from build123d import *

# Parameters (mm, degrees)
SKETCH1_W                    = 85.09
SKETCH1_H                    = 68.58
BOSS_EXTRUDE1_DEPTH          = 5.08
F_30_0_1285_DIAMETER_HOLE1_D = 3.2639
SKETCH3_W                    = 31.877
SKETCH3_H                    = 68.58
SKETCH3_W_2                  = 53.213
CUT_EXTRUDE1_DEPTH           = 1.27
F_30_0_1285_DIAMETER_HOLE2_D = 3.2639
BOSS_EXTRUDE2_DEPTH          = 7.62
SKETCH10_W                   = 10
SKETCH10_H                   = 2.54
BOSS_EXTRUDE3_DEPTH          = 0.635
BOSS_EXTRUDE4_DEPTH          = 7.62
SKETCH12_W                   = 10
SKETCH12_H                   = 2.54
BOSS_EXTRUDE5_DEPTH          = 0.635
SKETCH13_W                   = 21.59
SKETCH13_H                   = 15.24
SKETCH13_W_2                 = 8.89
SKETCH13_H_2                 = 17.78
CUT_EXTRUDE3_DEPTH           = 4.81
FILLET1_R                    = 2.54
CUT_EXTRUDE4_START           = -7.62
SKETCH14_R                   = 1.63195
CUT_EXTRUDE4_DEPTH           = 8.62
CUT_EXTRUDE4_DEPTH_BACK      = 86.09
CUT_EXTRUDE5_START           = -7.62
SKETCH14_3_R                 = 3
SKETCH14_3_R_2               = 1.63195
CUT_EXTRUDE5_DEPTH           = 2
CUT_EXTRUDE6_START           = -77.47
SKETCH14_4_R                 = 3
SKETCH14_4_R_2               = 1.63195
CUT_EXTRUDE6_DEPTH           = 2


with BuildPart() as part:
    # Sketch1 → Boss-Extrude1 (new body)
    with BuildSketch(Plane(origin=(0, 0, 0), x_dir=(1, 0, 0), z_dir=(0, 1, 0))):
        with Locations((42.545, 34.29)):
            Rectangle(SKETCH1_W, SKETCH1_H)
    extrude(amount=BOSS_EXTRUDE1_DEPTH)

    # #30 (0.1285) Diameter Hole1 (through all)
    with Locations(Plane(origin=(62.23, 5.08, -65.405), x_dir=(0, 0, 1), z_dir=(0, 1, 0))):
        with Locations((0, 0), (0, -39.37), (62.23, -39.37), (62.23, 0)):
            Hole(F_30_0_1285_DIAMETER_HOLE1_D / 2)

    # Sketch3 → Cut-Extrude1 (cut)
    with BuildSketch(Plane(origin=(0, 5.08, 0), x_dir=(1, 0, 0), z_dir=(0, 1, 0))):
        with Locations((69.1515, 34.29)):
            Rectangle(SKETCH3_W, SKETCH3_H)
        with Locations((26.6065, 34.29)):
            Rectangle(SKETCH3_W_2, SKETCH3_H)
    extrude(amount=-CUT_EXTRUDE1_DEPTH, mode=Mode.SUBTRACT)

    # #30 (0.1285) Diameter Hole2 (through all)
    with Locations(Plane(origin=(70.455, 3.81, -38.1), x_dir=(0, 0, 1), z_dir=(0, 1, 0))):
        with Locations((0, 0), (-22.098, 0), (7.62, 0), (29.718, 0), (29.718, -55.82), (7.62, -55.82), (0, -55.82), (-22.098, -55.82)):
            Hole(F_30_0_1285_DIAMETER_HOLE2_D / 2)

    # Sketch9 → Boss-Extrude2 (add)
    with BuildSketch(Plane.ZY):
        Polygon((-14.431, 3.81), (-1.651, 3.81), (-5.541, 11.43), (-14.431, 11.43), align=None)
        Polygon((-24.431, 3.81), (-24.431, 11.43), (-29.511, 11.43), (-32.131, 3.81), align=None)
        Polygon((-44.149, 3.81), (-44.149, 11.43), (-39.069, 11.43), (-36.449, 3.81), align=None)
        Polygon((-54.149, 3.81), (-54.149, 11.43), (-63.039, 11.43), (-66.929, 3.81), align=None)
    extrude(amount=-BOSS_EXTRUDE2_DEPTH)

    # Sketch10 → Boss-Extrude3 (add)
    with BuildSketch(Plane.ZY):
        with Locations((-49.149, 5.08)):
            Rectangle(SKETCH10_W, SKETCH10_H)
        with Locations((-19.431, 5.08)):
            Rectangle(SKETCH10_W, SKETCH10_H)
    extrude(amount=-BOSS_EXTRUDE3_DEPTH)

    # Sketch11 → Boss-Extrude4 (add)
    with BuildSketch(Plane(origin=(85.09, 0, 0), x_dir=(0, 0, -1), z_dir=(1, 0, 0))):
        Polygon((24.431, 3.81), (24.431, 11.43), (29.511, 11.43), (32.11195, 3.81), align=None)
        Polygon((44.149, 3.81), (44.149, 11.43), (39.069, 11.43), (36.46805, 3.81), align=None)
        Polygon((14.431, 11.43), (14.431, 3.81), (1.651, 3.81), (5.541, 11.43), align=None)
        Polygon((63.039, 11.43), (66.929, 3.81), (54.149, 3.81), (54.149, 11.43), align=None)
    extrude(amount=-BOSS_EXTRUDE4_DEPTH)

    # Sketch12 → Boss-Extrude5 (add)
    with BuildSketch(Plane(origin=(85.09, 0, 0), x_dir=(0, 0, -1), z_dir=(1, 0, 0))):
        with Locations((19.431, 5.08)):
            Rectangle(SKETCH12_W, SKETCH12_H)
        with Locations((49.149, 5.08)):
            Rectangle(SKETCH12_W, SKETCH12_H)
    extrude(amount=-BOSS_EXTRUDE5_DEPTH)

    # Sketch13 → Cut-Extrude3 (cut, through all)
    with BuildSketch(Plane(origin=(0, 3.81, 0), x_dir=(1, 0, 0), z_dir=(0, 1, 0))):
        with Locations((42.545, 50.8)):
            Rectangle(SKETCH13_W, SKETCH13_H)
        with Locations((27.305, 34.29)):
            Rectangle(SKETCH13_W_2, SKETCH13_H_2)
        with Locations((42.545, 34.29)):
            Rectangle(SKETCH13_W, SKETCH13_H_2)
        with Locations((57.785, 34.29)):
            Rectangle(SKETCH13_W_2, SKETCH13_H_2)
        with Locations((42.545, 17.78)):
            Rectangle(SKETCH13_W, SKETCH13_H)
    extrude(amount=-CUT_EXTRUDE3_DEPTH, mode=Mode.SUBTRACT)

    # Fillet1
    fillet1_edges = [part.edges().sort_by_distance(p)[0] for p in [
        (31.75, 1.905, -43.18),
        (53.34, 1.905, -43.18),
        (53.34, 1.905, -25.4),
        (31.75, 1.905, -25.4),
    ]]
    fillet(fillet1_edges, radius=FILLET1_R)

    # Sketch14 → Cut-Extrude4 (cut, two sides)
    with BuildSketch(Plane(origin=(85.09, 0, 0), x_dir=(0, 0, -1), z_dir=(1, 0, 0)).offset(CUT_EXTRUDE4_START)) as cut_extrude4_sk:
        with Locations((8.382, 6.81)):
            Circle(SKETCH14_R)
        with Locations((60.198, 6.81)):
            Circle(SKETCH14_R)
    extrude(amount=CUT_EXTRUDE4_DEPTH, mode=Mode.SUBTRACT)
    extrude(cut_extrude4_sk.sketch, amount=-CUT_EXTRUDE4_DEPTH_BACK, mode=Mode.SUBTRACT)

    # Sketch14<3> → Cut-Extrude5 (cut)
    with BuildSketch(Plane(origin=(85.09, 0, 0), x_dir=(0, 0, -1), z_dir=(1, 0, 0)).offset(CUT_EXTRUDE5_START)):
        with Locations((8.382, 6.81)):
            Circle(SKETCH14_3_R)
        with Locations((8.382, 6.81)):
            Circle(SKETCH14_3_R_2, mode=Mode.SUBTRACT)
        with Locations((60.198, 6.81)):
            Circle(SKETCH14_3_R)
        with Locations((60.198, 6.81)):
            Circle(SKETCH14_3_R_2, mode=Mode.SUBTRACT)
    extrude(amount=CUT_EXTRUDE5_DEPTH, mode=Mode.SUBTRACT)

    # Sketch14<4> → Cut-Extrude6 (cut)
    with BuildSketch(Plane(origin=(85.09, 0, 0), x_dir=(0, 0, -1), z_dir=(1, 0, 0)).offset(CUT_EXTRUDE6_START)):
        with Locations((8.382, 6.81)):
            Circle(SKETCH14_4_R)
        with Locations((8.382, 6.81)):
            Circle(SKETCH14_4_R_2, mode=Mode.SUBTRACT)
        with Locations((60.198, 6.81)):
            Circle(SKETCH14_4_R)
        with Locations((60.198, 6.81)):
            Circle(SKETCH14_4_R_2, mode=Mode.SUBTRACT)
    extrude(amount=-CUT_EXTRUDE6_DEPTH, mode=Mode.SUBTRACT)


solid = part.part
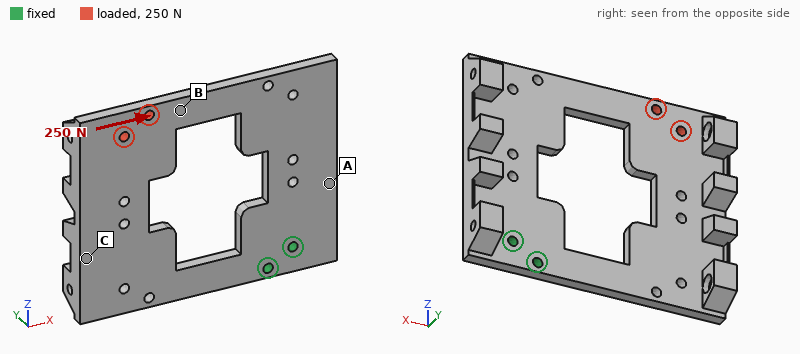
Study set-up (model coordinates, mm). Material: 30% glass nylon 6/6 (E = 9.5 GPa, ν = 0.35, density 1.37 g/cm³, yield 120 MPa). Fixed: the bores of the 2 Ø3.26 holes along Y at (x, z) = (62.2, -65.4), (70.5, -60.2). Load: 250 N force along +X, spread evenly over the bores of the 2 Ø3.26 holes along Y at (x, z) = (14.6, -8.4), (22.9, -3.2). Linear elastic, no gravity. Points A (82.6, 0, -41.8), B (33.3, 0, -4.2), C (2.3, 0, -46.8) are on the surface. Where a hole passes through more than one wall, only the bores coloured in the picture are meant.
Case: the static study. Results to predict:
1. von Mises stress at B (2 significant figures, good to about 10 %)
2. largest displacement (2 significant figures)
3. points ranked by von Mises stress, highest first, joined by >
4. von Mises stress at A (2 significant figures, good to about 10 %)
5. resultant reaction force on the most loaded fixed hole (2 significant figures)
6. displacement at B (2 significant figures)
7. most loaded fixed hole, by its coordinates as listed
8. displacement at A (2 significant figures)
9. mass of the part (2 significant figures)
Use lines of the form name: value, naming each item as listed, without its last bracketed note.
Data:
von Mises stress at B: 7.9 MPa
largest displacement: 0.81 mm
points ranked by von Mises stress, highest first, joined by >: A > B > C
von Mises stress at A: 16 MPa
resultant reaction force on the most loaded fixed hole: 1.2 kN
displacement at B: 0.61 mm
most loaded fixed hole, by its coordinates as listed: (70.5, -60.2)
displacement at A: 0.17 mm
mass of the part: 28 g
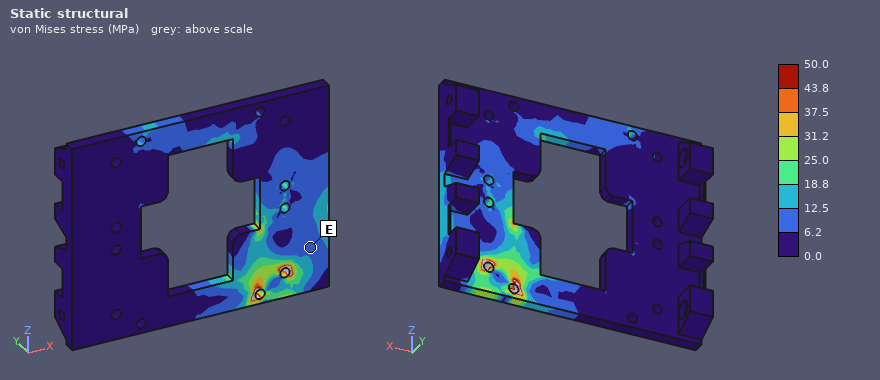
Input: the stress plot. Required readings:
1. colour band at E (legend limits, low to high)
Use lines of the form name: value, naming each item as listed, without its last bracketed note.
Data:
colour band at E: 6.2 to 12.5 MPa
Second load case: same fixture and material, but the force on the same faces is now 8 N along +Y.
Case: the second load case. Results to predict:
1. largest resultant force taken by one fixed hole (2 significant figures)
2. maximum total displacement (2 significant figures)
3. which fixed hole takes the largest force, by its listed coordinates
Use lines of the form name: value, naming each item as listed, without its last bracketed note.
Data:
largest resultant force taken by one fixed hole: 8.5 N
maximum total displacement: 1.1 mm
which fixed hole takes the largest force, by its listed coordinates: (62.2, -65.4)
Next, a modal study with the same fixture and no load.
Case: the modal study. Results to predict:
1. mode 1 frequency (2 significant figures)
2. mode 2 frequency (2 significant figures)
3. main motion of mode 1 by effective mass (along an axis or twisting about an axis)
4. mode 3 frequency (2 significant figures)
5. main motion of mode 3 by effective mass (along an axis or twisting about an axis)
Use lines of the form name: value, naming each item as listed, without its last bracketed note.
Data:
mode 1 frequency: 160 Hz
mode 2 frequency: 350 Hz
main motion of mode 1 by effective mass: along Y
mode 3 frequency: 670 Hz
main motion of mode 3 by effective mass: along Y
